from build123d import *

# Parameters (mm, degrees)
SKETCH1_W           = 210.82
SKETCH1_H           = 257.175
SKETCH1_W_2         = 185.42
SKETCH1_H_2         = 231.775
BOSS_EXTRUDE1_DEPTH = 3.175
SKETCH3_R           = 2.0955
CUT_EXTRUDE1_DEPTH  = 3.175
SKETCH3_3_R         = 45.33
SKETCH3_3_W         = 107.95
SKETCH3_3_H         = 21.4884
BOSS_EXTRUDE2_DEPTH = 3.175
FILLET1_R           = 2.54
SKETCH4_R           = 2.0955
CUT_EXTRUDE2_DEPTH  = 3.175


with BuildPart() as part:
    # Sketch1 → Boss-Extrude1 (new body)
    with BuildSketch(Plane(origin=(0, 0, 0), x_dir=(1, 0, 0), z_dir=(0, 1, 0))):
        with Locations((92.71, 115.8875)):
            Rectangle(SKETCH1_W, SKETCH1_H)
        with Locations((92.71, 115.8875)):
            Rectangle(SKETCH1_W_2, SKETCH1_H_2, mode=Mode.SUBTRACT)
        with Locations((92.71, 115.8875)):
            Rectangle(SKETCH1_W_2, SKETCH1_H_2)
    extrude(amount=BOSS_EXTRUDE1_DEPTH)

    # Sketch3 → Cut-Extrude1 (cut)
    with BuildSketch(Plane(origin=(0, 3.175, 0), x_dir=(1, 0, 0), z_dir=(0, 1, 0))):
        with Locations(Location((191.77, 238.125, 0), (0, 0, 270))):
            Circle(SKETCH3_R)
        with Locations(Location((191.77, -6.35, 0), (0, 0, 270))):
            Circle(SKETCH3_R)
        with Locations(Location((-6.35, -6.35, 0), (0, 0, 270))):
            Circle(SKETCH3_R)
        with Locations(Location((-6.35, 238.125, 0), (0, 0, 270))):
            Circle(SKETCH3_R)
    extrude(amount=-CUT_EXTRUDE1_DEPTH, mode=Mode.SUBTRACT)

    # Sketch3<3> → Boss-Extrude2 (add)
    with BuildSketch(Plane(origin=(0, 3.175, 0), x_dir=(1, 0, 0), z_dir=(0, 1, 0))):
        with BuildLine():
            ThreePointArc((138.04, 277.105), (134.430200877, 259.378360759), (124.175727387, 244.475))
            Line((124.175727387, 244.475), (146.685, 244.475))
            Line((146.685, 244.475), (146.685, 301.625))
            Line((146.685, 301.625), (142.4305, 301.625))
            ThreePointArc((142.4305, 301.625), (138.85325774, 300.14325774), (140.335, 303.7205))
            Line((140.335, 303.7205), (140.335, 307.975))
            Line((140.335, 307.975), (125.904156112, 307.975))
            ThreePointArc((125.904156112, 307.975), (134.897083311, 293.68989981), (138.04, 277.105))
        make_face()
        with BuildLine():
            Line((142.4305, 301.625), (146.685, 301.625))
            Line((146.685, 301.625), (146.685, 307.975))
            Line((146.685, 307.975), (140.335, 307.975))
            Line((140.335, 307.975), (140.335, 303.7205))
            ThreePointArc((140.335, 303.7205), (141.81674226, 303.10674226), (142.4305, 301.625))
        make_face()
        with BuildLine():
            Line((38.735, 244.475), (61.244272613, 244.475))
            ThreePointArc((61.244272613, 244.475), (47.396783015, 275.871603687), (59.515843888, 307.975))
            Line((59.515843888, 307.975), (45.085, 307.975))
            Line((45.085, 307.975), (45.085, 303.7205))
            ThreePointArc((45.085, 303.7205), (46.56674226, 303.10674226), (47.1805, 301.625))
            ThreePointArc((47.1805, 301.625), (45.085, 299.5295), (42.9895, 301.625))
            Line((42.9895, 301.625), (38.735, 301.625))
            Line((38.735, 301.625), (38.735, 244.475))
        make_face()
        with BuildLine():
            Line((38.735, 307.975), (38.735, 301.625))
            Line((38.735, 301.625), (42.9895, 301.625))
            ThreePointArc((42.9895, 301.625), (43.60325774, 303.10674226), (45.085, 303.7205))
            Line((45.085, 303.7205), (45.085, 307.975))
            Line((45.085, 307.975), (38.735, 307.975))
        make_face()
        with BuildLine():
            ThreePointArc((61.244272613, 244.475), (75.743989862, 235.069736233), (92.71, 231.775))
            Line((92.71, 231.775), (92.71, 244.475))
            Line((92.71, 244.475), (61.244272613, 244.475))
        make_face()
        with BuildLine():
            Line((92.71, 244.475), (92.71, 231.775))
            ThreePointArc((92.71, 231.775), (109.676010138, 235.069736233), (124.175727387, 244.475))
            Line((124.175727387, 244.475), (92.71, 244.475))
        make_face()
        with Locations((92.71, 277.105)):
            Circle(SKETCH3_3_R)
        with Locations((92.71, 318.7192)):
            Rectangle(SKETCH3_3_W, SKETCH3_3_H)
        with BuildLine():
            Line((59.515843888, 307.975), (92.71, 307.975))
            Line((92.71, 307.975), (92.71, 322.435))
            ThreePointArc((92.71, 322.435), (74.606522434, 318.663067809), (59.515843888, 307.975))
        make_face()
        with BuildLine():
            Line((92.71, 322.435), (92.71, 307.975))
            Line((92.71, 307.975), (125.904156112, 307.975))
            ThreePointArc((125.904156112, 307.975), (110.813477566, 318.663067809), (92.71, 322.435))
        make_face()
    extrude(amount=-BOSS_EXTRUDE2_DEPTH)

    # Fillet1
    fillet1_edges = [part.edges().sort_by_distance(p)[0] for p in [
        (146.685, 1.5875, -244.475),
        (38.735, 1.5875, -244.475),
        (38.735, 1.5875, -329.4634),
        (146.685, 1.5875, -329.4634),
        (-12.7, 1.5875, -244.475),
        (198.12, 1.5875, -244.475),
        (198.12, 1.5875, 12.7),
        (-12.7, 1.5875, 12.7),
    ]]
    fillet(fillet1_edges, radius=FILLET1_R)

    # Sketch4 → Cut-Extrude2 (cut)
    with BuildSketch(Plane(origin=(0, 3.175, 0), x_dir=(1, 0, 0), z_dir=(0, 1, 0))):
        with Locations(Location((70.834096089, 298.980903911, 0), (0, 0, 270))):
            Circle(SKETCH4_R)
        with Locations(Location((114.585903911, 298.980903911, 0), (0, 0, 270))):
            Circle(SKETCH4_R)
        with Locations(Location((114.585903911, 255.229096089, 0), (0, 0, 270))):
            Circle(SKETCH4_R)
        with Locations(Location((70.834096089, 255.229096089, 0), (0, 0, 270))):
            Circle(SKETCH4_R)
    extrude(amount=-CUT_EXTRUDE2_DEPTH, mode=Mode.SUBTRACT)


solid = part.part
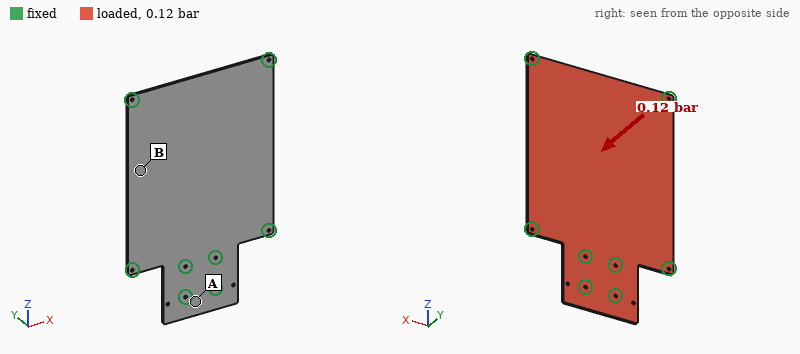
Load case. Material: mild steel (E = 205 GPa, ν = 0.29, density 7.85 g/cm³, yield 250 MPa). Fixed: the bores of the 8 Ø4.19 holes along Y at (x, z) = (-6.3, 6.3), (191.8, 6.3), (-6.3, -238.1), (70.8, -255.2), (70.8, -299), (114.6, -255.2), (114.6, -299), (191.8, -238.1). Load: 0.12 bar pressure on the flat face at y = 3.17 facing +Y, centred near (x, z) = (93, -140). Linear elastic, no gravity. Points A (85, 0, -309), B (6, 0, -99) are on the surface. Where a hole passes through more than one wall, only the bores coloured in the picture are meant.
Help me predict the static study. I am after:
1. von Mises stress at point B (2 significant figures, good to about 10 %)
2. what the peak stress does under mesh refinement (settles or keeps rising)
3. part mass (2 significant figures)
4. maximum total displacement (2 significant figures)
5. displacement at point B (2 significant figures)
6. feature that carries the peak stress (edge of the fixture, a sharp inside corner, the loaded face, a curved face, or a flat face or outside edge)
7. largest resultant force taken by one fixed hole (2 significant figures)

25 MPa
keeps rising
1.6 kg
0.41 mm
0.35 mm
edge of the fixture
150 N
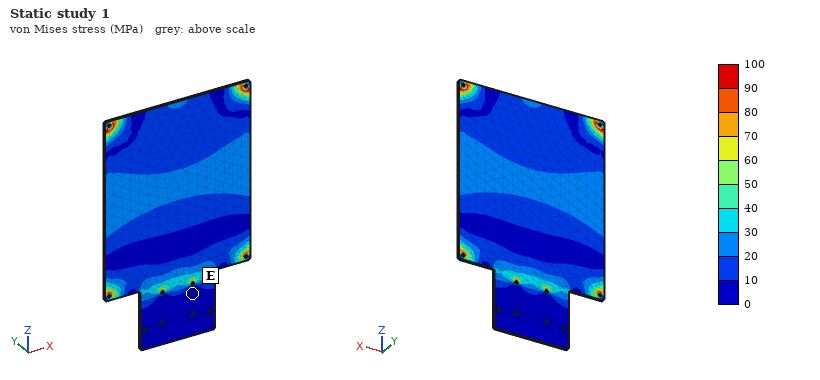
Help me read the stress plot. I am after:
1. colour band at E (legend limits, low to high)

0 to 10 MPa
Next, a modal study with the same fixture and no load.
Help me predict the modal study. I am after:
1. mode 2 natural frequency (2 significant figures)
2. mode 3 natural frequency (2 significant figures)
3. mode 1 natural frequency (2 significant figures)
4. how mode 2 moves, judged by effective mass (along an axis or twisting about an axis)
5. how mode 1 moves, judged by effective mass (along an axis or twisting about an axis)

320 Hz
410 Hz
200 Hz
twisting about Z
along Y
